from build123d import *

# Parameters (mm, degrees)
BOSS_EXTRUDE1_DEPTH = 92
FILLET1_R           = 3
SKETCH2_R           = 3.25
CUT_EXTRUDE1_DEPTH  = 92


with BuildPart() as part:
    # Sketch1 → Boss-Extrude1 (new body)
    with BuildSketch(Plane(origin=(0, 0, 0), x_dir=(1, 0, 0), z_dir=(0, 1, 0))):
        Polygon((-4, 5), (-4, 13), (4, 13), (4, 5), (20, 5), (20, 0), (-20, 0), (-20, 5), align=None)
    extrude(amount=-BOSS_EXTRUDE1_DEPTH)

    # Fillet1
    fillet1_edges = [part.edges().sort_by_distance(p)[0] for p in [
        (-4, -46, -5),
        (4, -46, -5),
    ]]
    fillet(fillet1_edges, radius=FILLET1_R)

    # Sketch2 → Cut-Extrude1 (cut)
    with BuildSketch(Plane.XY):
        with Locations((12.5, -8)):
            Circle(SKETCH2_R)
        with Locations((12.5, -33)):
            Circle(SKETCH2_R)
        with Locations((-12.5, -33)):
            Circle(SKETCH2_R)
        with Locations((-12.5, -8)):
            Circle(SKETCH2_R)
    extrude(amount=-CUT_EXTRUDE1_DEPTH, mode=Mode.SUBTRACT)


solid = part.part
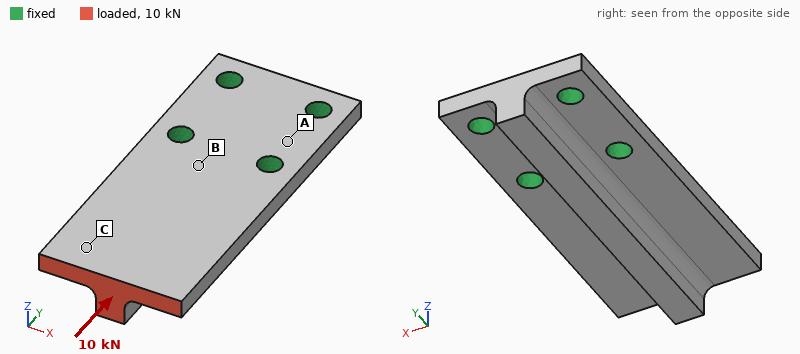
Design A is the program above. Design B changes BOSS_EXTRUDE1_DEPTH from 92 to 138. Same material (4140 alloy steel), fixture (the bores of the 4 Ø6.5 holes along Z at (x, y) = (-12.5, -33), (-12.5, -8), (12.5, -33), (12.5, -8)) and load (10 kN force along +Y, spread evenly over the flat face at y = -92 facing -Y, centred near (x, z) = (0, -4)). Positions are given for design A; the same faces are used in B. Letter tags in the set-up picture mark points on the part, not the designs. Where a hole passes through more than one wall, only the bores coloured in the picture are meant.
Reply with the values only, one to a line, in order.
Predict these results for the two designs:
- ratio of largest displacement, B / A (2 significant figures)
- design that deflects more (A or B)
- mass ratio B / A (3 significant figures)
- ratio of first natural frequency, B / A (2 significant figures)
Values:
1.7
B
1.51
0.35
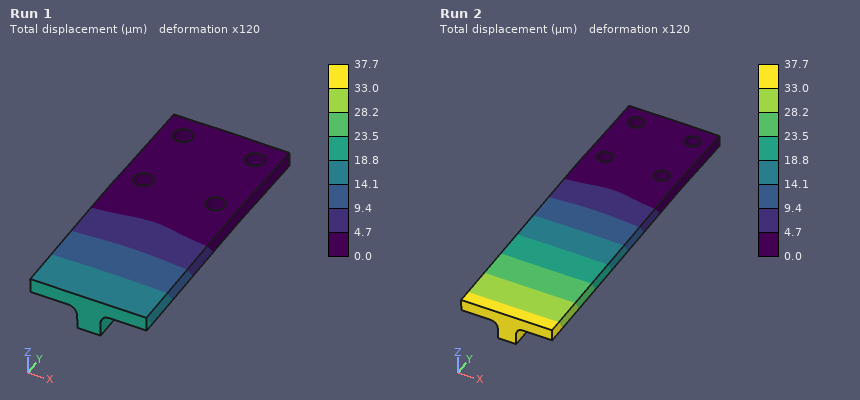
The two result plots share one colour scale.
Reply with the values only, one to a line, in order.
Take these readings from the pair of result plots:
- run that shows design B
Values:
Run 2
